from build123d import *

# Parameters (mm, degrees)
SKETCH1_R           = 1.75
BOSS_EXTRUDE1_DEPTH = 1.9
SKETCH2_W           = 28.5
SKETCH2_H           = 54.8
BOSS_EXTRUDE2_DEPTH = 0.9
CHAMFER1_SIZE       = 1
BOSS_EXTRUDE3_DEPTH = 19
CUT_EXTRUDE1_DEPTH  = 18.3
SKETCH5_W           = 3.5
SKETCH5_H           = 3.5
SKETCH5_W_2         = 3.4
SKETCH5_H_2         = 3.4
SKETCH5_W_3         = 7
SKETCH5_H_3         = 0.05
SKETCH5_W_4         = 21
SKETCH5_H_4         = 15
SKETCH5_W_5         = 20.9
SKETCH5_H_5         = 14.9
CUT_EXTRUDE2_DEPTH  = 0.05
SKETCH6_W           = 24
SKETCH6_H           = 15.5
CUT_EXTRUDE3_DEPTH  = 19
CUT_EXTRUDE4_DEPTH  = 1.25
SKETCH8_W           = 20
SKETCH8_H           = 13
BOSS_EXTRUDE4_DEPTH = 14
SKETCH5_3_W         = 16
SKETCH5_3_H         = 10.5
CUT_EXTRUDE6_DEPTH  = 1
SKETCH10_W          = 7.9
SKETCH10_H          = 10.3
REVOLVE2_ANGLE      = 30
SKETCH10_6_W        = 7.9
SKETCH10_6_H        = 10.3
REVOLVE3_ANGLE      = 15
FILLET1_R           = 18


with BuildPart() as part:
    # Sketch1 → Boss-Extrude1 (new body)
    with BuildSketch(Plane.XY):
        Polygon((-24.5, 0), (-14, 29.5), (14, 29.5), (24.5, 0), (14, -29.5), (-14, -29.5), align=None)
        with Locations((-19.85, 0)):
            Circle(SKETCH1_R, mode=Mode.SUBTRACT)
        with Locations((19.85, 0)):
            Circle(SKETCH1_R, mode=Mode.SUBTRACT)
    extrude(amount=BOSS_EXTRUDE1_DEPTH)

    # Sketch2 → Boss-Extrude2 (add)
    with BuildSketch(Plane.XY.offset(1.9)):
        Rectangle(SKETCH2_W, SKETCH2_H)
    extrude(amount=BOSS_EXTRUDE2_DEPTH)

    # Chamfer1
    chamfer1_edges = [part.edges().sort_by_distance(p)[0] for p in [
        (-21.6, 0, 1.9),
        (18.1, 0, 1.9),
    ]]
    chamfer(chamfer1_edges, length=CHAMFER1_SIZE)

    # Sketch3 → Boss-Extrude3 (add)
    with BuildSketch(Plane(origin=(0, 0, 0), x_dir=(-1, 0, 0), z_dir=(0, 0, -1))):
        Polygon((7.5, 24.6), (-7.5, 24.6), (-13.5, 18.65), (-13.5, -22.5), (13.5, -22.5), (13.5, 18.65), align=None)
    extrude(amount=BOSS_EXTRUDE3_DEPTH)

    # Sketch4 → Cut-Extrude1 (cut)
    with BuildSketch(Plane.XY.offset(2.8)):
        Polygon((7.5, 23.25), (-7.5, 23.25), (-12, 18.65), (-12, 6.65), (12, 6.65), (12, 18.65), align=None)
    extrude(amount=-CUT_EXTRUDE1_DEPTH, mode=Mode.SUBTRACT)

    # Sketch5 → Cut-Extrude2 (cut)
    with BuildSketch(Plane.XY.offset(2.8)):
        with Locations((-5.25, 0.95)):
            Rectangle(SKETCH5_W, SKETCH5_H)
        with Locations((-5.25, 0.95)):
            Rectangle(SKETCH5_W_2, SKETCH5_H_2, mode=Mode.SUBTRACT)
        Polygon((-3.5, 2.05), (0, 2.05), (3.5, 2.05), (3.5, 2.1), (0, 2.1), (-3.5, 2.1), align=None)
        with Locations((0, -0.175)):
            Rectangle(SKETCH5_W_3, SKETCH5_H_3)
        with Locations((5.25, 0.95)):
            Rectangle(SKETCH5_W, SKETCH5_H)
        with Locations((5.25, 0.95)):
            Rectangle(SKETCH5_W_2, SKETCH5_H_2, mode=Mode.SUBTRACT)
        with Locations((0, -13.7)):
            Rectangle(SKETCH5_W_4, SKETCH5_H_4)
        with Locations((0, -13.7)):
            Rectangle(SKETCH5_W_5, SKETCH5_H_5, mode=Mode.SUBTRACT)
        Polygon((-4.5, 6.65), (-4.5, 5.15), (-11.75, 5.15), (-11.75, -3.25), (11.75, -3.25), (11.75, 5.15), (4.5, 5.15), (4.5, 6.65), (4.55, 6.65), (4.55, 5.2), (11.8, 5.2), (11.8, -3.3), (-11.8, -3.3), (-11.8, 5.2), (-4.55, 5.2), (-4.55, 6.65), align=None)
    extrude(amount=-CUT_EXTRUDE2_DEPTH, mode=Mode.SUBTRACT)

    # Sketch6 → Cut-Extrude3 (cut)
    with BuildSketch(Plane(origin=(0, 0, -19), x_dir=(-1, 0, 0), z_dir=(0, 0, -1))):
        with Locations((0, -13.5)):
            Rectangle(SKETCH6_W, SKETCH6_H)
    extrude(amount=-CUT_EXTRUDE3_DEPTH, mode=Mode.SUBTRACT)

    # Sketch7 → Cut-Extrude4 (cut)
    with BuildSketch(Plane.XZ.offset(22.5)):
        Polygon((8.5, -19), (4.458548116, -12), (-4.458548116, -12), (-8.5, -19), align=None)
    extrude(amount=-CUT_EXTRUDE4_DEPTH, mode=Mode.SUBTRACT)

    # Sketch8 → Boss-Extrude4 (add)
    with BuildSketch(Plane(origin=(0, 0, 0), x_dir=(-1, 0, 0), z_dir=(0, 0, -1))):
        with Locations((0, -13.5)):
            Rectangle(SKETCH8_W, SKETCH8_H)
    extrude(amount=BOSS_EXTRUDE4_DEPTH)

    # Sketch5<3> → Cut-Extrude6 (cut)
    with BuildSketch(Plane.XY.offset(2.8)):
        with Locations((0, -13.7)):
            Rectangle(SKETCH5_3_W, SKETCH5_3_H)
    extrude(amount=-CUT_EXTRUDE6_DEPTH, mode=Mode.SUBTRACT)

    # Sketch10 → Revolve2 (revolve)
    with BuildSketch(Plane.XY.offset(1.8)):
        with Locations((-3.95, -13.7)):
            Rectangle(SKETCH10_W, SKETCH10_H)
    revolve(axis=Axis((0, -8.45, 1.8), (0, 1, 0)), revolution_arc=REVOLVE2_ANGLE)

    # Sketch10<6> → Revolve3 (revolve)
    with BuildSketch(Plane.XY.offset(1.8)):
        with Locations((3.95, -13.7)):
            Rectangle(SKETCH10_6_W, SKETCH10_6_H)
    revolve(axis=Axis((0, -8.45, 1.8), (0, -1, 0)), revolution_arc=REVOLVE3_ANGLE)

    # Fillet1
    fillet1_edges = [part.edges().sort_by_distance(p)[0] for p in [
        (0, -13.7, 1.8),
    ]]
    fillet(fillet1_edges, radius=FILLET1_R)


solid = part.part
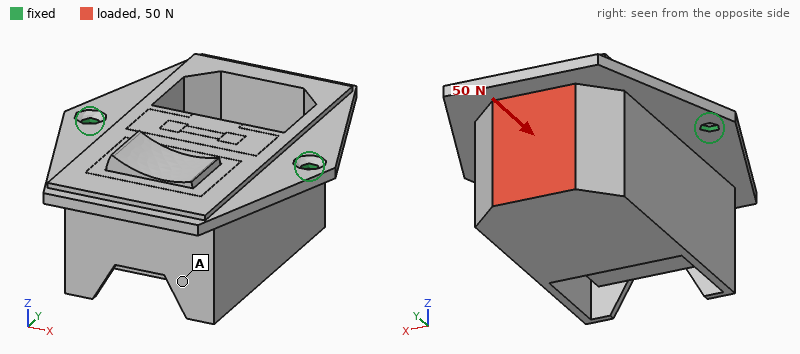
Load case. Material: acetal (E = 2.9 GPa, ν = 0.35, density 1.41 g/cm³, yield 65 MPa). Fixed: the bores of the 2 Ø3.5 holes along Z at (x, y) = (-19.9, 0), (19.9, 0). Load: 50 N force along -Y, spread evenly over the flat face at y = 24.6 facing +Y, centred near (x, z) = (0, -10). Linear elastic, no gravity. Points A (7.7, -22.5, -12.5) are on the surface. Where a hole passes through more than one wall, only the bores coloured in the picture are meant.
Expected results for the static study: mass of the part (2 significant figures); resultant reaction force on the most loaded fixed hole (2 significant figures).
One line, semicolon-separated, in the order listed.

27 g; 25 N
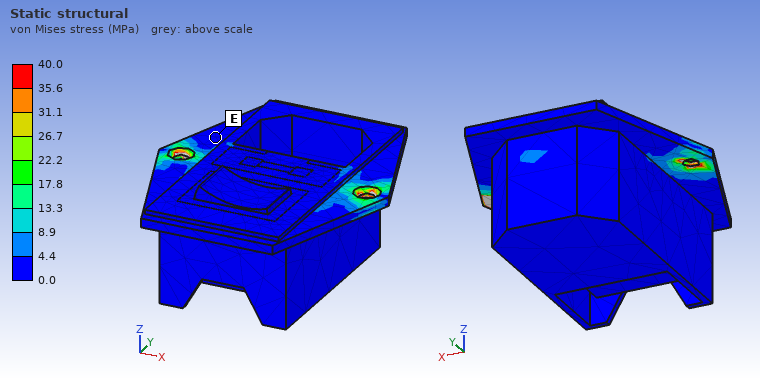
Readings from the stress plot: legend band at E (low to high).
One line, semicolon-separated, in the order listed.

0.0 to 4.4 MPa
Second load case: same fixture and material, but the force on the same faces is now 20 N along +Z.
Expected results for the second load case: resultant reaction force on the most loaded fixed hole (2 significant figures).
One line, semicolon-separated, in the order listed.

10 N
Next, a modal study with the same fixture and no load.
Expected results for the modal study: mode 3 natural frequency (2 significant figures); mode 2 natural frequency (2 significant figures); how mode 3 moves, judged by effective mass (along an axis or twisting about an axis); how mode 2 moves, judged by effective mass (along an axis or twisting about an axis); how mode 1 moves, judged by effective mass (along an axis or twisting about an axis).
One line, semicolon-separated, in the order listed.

1300 Hz; 1100 Hz; along X; along Z; along Y
